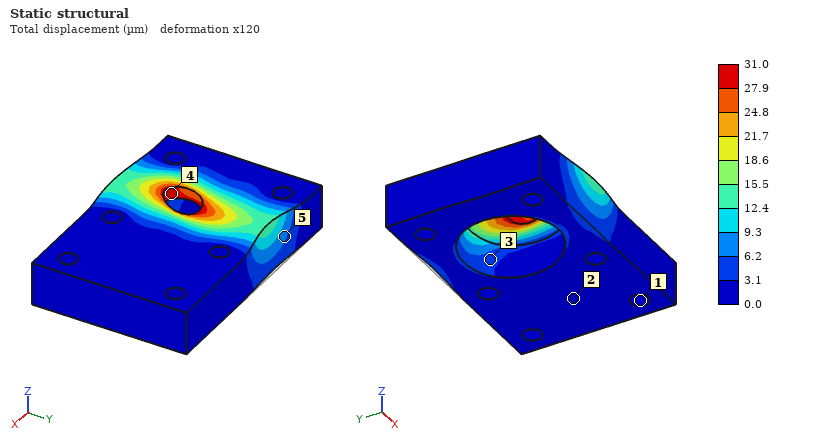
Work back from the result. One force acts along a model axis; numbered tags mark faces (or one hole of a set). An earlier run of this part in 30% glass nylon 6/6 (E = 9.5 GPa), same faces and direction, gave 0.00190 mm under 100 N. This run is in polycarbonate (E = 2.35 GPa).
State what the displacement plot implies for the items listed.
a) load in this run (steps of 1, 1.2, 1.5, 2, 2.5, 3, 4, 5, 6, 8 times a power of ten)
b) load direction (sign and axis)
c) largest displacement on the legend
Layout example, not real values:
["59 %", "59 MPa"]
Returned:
["400 N", "-Y", "31.0 µm"]
